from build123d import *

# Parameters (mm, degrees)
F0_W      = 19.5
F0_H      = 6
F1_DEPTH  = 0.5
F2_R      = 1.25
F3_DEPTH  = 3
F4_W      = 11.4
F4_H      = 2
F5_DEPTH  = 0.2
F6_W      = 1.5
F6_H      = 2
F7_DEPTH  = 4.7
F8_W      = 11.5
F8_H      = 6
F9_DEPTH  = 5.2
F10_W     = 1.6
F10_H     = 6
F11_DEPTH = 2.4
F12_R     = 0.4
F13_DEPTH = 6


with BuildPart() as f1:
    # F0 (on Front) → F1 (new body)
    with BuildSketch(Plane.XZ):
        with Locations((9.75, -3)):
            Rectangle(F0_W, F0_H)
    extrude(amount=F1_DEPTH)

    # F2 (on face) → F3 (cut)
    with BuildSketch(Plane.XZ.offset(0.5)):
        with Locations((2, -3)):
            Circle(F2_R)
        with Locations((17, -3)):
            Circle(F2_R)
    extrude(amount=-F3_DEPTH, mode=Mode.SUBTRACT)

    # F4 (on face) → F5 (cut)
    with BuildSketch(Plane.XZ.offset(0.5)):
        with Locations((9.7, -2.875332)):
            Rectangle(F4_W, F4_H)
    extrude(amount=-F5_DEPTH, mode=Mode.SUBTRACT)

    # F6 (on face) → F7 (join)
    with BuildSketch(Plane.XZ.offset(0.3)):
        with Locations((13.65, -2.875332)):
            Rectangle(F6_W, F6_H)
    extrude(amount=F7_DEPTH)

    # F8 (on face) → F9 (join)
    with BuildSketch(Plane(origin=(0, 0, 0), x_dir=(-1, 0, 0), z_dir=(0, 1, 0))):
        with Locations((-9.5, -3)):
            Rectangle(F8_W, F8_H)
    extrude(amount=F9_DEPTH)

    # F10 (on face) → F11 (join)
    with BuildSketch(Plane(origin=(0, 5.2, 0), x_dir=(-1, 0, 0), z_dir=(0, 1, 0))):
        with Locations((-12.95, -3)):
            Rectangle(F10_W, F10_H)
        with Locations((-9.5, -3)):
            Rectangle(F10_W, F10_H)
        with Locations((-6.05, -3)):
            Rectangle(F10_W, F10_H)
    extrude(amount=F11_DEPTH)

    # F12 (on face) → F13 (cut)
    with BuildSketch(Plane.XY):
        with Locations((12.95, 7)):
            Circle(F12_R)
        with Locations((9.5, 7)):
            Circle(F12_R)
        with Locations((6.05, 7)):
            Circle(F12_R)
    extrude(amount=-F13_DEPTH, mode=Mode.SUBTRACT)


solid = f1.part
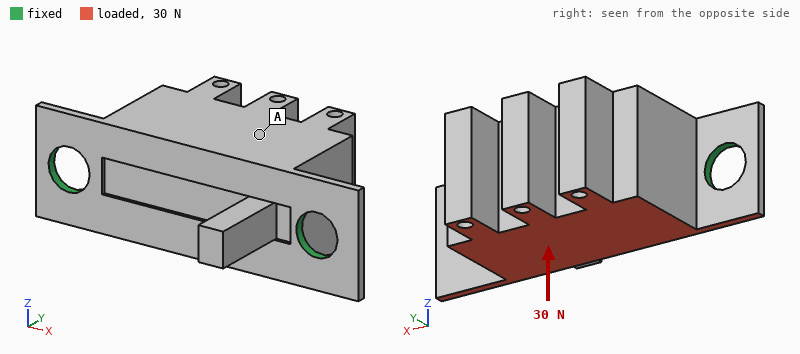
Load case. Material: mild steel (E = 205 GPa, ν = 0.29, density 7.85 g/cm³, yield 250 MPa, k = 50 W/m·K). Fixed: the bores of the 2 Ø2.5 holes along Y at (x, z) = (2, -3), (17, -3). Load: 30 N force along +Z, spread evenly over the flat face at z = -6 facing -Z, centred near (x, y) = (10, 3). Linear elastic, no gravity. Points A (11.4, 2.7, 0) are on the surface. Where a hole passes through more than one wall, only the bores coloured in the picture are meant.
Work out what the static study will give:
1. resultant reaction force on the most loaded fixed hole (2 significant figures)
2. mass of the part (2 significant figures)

15 N
3.8 g
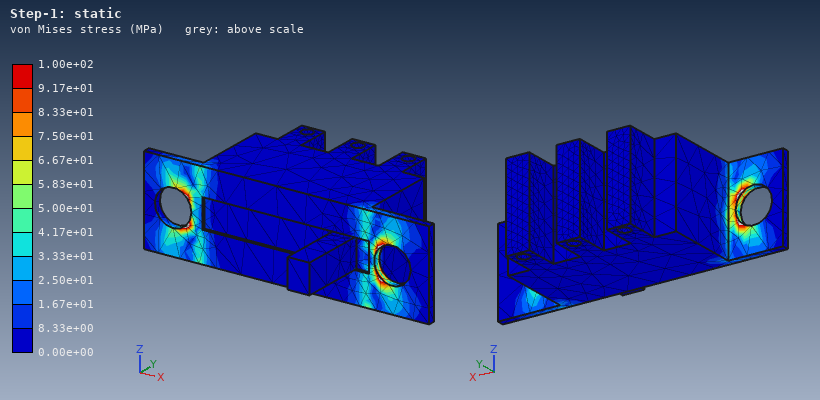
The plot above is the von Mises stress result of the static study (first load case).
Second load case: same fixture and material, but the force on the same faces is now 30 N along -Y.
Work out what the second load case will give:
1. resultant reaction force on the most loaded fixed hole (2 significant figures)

18 N
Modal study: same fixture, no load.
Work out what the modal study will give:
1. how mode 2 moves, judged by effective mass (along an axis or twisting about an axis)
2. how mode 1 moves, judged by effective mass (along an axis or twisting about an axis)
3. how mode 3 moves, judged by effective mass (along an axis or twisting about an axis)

along Y
along Z
along X
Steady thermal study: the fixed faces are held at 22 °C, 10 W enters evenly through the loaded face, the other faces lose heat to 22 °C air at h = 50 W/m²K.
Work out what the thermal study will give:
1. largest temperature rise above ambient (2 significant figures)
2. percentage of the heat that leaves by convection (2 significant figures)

66 K
13 %
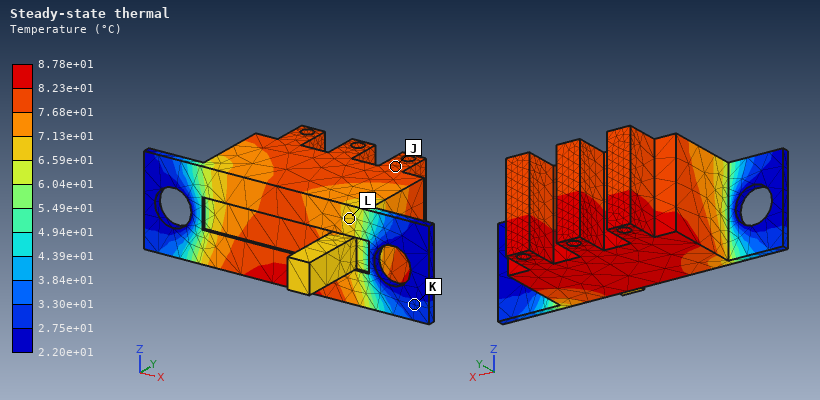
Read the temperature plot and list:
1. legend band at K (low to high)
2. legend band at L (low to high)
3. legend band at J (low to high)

2.75e+01 to 3.30e+01 °C
6.59e+01 to 7.13e+01 °C
7.68e+01 to 8.23e+01 °C
